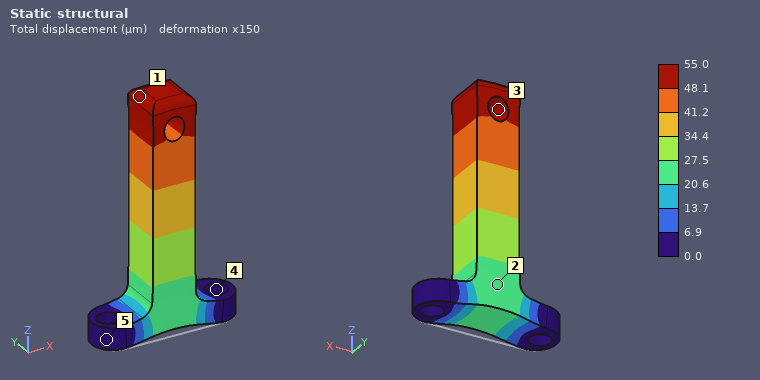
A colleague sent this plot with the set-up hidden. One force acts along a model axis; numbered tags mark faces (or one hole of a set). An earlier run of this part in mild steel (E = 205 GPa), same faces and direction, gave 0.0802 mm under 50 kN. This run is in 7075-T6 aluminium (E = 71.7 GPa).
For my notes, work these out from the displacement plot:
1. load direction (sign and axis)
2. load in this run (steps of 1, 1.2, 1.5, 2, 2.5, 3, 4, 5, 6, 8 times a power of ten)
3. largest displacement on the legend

+Z
12 kN
55.0 µm
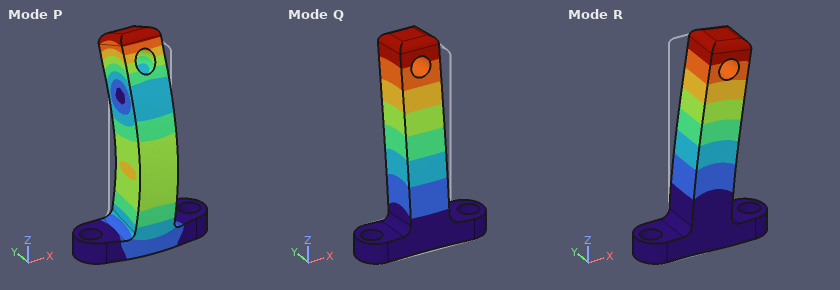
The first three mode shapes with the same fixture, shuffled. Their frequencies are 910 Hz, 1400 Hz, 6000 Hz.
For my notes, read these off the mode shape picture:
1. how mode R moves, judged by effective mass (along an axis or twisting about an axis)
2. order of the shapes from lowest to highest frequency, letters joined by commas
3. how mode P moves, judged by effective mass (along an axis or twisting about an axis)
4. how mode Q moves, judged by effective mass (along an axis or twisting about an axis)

along X
Q, R, P
along Y
along Y
